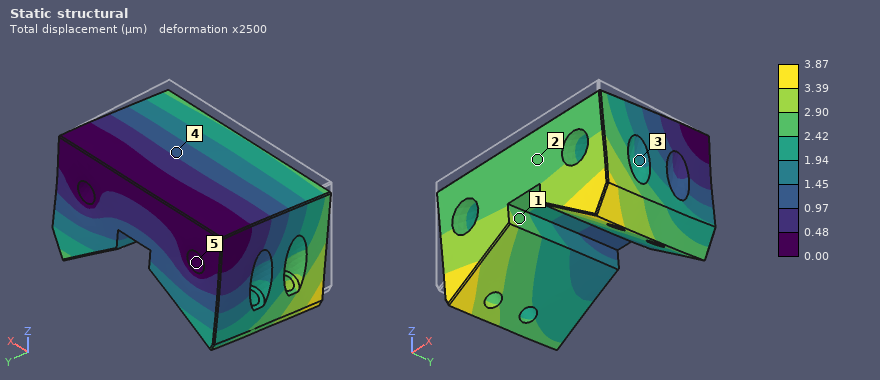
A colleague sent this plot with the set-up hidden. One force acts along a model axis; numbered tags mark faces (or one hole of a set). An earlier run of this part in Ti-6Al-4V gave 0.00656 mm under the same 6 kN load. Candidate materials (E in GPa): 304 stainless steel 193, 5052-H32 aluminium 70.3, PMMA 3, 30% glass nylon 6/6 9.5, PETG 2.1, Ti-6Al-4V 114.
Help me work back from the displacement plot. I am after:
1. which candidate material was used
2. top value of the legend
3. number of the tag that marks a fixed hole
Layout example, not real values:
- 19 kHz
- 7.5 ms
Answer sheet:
- 304 stainless steel
- 3.87 µm
- 5
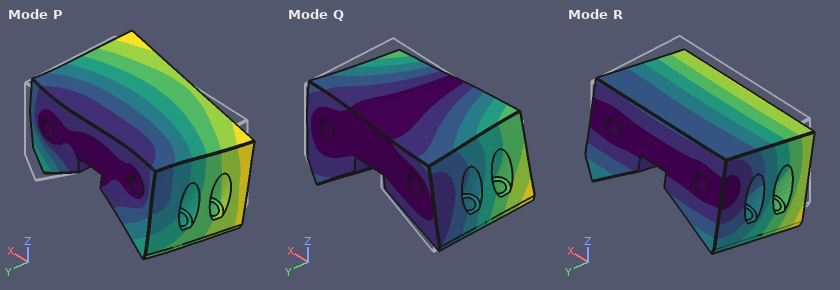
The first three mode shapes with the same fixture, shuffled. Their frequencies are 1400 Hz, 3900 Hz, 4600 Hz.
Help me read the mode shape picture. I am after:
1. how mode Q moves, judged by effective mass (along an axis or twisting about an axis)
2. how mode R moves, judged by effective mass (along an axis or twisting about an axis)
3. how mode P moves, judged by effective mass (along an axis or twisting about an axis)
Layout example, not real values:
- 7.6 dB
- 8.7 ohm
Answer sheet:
- along X
- along Z
- along X
